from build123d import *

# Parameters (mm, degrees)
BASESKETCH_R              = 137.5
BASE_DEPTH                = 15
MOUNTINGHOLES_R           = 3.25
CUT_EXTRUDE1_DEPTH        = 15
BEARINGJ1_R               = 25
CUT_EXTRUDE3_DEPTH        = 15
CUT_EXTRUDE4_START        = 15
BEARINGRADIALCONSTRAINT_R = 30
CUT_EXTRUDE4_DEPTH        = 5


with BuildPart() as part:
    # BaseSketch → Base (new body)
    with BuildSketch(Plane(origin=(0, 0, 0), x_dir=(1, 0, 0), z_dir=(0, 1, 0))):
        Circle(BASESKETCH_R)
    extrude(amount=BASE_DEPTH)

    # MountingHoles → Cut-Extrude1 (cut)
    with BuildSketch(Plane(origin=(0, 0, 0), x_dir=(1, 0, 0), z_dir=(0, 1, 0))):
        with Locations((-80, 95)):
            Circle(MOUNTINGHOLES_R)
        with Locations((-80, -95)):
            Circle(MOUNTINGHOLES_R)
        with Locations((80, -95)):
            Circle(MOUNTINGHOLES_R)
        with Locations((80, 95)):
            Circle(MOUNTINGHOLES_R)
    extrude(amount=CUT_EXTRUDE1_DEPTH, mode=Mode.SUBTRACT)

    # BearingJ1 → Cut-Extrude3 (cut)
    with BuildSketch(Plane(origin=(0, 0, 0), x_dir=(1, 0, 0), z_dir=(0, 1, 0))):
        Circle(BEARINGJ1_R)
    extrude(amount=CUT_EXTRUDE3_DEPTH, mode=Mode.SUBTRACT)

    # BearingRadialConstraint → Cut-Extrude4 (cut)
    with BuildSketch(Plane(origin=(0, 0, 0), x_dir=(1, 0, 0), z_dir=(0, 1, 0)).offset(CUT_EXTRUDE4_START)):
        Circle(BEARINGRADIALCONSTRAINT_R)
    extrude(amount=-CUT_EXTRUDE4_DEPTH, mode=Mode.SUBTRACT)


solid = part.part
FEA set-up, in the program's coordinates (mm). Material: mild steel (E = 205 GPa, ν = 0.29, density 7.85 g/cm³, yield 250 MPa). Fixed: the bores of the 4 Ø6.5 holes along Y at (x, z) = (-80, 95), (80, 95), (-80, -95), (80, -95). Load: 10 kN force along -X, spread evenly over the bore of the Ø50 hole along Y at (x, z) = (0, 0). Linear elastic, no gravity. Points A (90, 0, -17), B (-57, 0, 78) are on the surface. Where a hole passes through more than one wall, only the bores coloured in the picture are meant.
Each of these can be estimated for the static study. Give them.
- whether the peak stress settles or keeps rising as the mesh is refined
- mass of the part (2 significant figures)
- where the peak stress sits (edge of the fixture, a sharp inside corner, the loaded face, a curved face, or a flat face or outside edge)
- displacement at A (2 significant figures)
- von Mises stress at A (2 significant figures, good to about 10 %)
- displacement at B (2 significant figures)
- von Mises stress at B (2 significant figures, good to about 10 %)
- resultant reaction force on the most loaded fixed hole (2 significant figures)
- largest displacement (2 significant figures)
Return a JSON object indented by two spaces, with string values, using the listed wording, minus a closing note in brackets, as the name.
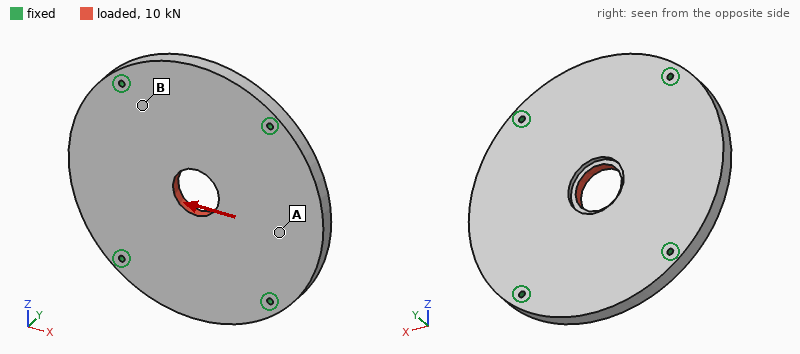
{
  "whether the peak stress settles or keeps rising as the mesh is refined": "keeps rising",
  "mass of the part": "6.7 kg",
  "where the peak stress sits": "edge of the fixture",
  "displacement at A": "2.0 µm",
  "von Mises stress at A": "1.3 MPa",
  "displacement at B": "0.81 µm",
  "von Mises stress at B": "4.0 MPa",
  "resultant reaction force on the most loaded fixed hole": "2.6 kN",
  "largest displacement": "3.0 µm"
}
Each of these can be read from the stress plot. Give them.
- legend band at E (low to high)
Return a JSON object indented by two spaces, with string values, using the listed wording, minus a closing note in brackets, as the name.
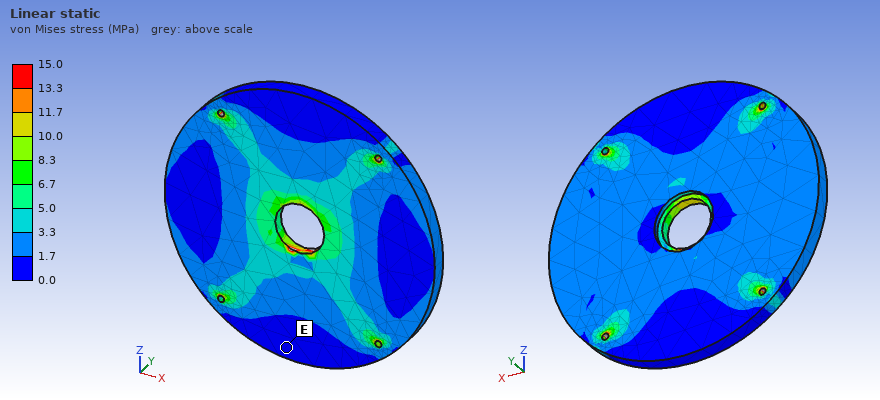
{
  "legend band at E": "0.0 to 1.7 MPa"
}
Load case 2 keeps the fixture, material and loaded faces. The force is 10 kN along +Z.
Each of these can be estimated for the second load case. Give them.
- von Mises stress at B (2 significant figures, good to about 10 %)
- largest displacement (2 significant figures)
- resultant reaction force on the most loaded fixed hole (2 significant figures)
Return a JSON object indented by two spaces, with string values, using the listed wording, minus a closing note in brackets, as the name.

{
  "von Mises stress at B": "3.5 MPa",
  "largest displacement": "2.7 µm",
  "resultant reaction force on the most loaded fixed hole": "2.6 kN"
}
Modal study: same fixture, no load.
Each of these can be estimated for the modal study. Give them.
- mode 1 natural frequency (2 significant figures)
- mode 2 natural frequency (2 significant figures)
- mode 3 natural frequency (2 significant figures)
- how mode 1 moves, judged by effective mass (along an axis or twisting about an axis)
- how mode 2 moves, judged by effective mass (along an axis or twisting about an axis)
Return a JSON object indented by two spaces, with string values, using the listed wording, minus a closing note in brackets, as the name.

{
  "mode 1 natural frequency": "1400 Hz",
  "mode 2 natural frequency": "1600 Hz",
  "mode 3 natural frequency": "1800 Hz",
  "how mode 1 moves, judged by effective mass": "along Y",
  "how mode 2 moves, judged by effective mass": "twisting about Z"
}
